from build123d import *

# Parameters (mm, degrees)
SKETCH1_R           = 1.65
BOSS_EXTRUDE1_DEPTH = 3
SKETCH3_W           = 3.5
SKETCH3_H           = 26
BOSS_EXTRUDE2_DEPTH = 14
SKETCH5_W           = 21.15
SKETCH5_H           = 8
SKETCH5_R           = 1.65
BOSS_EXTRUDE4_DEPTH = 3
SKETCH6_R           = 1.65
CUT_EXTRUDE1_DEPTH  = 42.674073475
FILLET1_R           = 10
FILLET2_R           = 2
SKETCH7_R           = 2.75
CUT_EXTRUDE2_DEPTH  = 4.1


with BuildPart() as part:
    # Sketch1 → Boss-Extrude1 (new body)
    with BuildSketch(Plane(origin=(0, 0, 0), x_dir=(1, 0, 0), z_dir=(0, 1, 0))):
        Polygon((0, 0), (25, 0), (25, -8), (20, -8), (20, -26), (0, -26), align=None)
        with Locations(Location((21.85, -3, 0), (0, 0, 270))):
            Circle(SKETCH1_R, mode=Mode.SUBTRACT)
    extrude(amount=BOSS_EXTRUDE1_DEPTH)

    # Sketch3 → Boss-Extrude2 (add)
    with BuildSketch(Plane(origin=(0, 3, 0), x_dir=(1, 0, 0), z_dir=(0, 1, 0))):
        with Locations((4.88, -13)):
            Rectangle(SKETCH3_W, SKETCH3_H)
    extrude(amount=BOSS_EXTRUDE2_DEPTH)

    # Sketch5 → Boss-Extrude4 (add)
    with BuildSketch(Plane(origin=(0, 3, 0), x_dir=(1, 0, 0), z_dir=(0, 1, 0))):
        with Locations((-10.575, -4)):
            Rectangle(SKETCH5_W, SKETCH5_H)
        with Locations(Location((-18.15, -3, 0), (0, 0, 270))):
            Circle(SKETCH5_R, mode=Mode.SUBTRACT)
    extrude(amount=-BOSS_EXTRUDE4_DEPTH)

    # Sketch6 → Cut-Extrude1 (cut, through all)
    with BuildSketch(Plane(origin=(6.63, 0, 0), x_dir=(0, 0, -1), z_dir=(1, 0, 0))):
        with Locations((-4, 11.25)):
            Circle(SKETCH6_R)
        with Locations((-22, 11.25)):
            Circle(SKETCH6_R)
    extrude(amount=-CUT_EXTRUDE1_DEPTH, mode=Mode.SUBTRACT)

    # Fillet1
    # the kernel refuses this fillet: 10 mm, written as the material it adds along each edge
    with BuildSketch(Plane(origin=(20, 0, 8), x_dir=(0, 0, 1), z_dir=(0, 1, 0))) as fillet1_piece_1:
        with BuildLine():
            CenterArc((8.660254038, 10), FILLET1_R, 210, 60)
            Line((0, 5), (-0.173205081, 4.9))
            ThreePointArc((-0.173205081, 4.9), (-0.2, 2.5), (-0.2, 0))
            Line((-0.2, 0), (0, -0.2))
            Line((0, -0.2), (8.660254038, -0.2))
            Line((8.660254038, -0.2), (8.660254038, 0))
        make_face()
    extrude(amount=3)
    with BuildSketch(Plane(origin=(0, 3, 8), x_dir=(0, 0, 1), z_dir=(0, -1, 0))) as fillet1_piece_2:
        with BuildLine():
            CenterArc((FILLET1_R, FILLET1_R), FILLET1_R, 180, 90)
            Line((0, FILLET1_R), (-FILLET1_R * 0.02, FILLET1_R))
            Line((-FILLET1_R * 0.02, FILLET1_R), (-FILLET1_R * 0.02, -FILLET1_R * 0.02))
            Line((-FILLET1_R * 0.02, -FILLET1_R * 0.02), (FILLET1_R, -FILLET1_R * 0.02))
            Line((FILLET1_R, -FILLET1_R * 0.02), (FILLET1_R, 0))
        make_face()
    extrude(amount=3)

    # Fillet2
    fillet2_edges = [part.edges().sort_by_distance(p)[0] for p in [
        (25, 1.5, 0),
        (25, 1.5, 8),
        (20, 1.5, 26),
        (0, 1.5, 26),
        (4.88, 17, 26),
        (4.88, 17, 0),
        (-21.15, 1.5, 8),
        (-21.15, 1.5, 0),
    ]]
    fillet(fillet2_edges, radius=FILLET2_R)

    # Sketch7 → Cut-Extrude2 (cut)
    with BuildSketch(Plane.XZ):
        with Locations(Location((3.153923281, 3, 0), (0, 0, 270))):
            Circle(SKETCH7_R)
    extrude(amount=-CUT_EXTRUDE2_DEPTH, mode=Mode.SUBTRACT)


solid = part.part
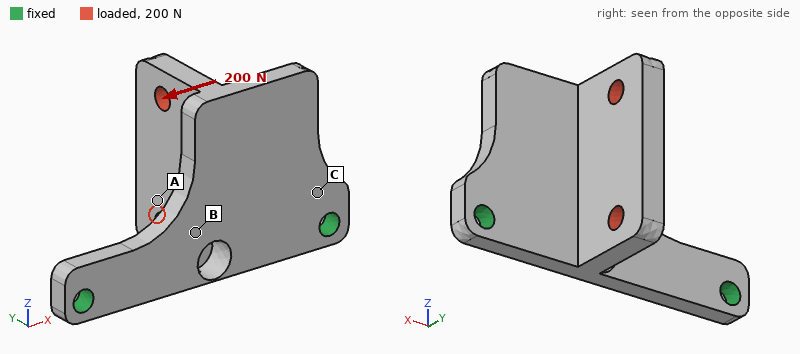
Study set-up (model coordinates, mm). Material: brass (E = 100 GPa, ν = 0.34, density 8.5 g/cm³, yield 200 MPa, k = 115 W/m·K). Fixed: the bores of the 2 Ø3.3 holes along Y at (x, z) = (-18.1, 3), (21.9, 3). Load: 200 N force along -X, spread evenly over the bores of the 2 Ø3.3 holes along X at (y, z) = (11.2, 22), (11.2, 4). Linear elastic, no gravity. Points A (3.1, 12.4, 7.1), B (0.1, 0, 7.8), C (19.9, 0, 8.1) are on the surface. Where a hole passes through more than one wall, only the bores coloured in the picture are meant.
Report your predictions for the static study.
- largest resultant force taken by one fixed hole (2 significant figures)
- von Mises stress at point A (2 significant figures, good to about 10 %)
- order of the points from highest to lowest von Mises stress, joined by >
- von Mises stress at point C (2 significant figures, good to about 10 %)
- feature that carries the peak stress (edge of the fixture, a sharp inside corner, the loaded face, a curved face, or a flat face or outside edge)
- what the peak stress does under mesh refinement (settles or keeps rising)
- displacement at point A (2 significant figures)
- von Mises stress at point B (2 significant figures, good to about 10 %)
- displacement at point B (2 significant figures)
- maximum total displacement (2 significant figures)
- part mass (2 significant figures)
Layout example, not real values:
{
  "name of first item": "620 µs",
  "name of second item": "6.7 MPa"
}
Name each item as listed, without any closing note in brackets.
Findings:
{
  "largest resultant force taken by one fixed hole": "130 N",
  "von Mises stress at point A": "5.0 MPa",
  "order of the points from highest to lowest von Mises stress, joined by >": "B > C > A",
  "von Mises stress at point C": "13 MPa",
  "feature that carries the peak stress": "a sharp inside corner",
  "what the peak stress does under mesh refinement": "keeps rising",
  "displacement at point A": "33 µm",
  "von Mises stress at point B": "40 MPa",
  "displacement at point B": "17 µm",
  "maximum total displacement": "52 µm",
  "part mass": "28 g"
}
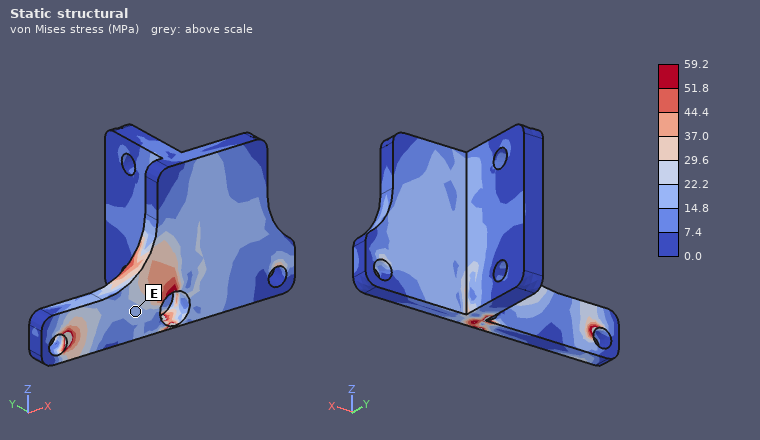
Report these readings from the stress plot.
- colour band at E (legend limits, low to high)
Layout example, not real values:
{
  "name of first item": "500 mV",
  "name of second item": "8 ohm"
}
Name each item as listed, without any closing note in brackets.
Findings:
{
  "colour band at E": "14.8 to 22.2 MPa"
}
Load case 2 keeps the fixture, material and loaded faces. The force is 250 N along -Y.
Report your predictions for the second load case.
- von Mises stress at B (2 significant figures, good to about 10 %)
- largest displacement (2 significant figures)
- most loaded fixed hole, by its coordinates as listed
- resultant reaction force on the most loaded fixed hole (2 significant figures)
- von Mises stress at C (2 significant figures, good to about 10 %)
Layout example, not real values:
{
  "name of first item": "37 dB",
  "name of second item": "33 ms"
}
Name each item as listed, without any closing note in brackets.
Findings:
{
  "von Mises stress at B": "62 MPa",
  "largest displacement": "0.14 mm",
  "most loaded fixed hole, by its coordinates as listed": "(21.9, 3)",
  "resultant reaction force on the most loaded fixed hole": "150 N",
  "von Mises stress at C": "74 MPa"
}
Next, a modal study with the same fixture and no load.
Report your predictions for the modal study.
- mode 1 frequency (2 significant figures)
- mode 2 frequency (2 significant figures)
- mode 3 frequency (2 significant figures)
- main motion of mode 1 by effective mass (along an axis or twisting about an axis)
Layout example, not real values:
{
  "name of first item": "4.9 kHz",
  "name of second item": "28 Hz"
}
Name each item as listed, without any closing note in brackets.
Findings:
{
  "mode 1 frequency": "1700 Hz",
  "mode 2 frequency": "3600 Hz",
  "mode 3 frequency": "5200 Hz",
  "main motion of mode 1 by effective mass": "along Y"
}
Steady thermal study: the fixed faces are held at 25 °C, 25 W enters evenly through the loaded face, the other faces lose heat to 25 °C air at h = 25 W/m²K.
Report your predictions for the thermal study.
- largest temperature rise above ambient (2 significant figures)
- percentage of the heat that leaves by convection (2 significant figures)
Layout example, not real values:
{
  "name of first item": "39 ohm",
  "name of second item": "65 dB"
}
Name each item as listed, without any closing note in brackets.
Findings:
{
  "largest temperature rise above ambient": "82 K",
  "percentage of the heat that leaves by convection": "12 %"
}
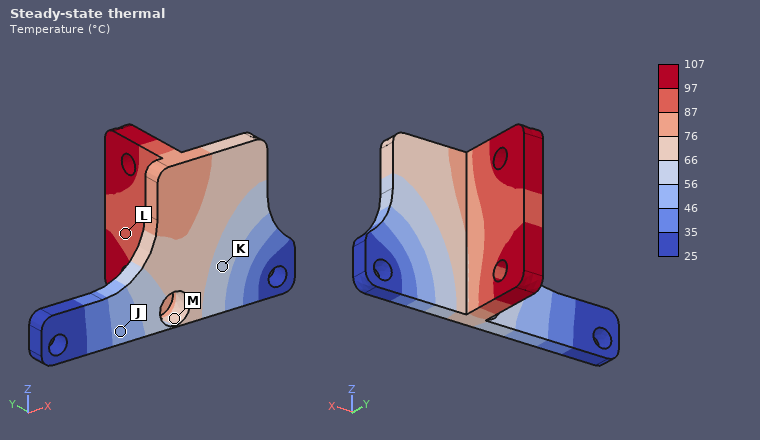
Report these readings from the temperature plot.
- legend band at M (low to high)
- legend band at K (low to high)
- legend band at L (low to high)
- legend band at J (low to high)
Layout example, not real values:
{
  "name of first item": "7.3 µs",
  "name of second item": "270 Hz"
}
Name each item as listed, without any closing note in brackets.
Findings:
{
  "legend band at M": "66 to 76 °C",
  "legend band at K": "56 to 66 °C",
  "legend band at L": "87 to 97 °C",
  "legend band at J": "46 to 56 °C"
}
